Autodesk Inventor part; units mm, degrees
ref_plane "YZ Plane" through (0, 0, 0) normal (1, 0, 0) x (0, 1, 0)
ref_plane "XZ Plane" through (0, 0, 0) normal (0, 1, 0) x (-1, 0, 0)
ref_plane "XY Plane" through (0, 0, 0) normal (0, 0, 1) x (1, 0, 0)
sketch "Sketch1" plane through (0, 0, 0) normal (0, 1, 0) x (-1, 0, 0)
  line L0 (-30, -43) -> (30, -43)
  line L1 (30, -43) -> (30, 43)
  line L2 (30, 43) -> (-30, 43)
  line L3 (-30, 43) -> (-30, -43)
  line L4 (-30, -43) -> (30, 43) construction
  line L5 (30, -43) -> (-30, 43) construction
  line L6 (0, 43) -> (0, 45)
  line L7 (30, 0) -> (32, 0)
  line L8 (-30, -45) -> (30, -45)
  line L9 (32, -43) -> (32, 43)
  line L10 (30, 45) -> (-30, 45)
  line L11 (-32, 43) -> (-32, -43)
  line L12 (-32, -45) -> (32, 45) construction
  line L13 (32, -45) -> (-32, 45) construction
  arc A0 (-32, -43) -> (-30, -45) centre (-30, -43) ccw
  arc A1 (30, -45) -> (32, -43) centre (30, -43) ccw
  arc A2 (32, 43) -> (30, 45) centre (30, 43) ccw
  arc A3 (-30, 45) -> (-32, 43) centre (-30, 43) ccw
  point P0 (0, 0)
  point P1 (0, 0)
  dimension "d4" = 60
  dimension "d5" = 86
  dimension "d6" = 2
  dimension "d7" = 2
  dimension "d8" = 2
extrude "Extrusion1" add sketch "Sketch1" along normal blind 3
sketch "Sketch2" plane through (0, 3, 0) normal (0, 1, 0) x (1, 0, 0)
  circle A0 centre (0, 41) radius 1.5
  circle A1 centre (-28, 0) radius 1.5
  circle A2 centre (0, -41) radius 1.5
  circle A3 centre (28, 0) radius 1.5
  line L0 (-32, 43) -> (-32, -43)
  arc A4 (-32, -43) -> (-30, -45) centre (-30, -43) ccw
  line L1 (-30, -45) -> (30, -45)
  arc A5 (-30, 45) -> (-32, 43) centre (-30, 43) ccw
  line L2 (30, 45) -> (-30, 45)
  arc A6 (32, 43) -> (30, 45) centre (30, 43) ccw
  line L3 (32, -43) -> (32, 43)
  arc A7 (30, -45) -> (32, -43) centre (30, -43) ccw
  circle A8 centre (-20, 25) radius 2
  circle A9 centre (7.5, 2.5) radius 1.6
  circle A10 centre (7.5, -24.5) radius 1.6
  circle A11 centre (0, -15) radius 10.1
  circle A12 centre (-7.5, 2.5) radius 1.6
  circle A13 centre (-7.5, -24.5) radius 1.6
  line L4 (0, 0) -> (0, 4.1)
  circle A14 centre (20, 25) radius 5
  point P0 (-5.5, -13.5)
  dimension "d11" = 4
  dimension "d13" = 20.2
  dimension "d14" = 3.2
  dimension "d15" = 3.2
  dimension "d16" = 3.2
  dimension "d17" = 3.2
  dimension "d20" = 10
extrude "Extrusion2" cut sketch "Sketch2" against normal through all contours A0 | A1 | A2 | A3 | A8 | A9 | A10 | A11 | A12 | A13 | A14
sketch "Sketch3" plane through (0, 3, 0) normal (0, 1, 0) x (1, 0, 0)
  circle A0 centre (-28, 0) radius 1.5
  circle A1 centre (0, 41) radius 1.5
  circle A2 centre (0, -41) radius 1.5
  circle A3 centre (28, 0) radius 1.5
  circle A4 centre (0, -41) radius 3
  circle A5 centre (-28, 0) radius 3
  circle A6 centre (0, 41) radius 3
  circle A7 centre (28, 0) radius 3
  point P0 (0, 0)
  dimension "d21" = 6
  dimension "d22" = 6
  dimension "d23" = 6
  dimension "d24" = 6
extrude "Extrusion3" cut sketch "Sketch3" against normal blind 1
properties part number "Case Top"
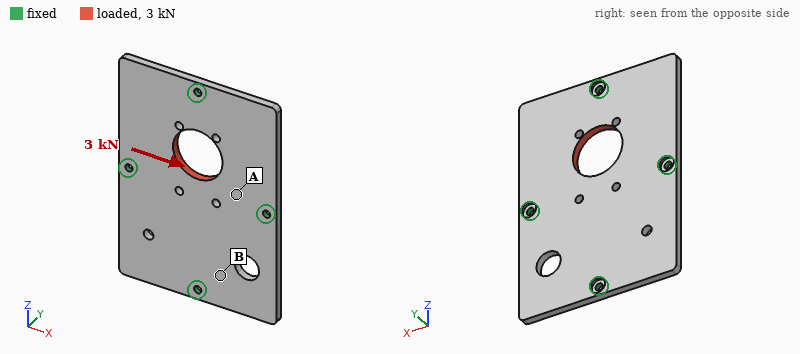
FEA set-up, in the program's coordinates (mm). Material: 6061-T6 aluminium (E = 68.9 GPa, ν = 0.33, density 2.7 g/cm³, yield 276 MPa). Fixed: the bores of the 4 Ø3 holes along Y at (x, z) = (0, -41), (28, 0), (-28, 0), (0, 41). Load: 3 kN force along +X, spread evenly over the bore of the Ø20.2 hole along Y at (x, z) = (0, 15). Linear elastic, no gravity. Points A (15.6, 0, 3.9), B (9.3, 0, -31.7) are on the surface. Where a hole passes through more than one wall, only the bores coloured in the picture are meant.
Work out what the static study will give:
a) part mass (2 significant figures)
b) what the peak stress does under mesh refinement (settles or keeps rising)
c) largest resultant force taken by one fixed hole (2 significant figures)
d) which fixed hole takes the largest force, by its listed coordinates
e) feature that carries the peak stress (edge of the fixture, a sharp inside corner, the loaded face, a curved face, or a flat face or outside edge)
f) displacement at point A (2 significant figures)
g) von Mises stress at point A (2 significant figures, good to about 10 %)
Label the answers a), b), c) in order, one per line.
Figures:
a) 43 g
b) keeps rising
c) 1.1 kN
d) (0, 41)
e) edge of the fixture
f) 6.0 µm
g) 20 MPa
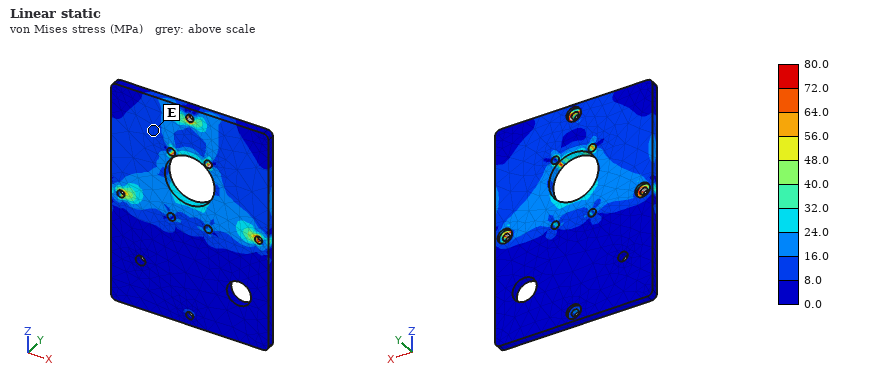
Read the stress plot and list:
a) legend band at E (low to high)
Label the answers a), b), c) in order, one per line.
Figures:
a) 8.0 to 16.0 MPa
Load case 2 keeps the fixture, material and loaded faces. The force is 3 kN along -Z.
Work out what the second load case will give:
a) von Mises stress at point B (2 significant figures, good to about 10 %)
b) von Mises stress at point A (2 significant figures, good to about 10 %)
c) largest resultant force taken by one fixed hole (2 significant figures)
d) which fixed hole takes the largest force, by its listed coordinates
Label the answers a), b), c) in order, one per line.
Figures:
a) 7.2 MPa
b) 10 MPa
c) 910 N
d) (0, 41)
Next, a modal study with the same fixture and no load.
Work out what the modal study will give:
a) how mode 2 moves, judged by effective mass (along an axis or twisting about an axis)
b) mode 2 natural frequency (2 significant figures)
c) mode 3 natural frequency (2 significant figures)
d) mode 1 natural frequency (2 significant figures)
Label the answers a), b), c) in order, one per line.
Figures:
a) twisting about Z
b) 2900 Hz
c) 3200 Hz
d) 2700 Hz
